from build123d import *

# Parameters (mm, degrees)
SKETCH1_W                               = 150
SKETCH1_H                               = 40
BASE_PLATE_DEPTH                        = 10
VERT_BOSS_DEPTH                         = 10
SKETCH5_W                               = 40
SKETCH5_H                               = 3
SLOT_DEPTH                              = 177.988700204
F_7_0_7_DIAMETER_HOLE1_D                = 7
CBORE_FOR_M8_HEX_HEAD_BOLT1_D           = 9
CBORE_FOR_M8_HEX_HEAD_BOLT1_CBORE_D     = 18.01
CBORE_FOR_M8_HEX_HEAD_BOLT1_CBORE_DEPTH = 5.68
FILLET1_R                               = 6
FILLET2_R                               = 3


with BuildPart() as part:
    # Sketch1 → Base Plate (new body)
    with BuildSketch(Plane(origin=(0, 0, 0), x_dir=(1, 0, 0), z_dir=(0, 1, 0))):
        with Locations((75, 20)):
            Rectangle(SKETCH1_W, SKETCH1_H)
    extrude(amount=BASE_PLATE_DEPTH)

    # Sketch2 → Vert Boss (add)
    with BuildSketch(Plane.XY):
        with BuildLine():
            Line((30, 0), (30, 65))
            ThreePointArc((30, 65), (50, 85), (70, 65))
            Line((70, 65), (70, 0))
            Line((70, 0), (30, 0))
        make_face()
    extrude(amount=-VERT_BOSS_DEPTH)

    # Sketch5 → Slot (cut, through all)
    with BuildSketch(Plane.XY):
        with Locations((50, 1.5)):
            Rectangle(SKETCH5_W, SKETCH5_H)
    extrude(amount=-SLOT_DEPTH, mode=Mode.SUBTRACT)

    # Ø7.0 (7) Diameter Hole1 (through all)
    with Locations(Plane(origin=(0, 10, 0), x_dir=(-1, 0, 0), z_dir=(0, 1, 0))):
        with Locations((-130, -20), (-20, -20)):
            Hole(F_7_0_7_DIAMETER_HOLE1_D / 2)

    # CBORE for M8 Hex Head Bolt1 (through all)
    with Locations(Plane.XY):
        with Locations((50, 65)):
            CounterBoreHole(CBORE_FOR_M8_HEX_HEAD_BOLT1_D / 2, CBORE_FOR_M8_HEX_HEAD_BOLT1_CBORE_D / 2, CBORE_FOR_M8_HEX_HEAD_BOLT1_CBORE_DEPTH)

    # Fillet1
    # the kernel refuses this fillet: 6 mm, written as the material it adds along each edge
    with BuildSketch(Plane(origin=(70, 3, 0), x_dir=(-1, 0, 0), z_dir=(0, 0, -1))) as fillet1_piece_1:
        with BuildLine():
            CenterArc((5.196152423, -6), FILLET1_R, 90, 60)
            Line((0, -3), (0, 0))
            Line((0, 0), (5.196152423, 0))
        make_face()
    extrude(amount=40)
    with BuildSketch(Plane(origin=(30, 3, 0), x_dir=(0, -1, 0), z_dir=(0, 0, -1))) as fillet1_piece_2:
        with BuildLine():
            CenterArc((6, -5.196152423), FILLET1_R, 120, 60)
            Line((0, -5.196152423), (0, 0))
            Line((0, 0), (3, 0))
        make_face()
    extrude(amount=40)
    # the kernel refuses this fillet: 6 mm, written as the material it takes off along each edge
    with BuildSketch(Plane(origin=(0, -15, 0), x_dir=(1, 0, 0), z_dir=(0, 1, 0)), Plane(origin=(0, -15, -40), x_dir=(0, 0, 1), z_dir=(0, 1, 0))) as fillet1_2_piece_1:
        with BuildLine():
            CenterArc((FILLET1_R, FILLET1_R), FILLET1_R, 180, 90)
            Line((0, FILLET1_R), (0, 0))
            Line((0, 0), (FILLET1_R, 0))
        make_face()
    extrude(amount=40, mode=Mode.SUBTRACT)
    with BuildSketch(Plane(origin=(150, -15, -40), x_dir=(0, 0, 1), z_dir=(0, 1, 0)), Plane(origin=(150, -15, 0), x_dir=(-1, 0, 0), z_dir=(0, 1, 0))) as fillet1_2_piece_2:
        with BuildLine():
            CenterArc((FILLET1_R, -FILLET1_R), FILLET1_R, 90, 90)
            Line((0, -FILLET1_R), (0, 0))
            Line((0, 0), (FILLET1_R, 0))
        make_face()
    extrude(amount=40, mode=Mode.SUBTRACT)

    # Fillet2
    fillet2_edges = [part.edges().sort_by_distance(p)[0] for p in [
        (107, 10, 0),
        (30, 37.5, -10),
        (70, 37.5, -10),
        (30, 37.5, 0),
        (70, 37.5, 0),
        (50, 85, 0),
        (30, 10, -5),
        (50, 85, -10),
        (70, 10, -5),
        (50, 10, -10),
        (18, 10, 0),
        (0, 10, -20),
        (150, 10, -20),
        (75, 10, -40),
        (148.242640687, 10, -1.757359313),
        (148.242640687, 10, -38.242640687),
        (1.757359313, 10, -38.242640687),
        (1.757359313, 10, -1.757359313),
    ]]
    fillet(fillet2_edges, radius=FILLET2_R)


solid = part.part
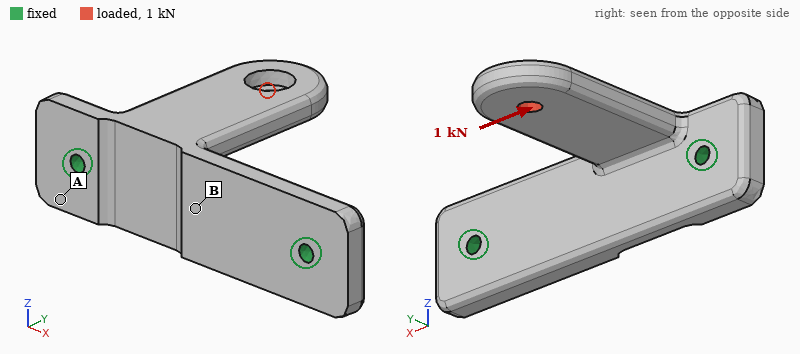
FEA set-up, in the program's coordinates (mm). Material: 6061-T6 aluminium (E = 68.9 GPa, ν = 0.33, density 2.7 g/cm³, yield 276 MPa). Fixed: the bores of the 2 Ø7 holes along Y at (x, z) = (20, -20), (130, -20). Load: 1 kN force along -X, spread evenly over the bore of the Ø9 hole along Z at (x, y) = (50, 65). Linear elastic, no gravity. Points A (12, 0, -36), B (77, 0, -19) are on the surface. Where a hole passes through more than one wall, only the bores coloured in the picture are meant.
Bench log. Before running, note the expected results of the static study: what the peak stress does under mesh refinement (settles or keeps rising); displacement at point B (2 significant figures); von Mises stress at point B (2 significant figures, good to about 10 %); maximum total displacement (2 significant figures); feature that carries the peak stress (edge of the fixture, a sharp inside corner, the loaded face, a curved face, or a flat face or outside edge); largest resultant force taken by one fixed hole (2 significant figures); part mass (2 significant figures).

keeps rising
0.052 mm
21 MPa
0.21 mm
a sharp inside corner
820 N
220 g
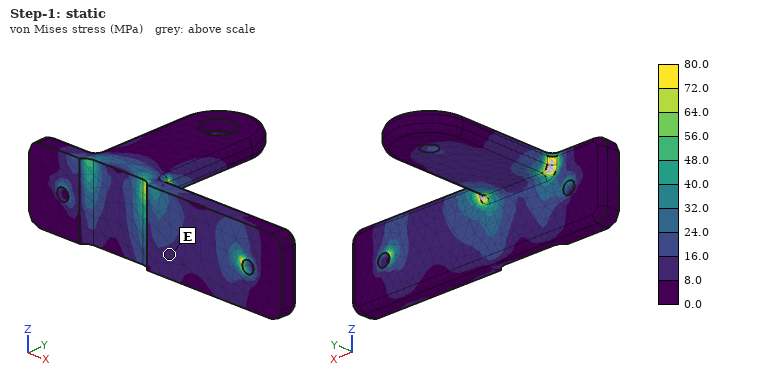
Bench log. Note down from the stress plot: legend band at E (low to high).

8.0 to 16.0 MPa
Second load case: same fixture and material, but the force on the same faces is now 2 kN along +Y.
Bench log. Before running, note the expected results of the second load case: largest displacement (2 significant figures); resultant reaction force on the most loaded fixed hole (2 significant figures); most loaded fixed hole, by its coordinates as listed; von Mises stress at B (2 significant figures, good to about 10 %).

0.11 mm
1.6 kN
(20, -20)
15 MPa
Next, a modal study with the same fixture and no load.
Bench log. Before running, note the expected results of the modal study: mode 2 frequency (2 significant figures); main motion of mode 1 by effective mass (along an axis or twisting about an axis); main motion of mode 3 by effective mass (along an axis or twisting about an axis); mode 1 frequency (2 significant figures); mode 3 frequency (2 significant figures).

1900 Hz
along Z
along Y
1100 Hz
4500 Hz
